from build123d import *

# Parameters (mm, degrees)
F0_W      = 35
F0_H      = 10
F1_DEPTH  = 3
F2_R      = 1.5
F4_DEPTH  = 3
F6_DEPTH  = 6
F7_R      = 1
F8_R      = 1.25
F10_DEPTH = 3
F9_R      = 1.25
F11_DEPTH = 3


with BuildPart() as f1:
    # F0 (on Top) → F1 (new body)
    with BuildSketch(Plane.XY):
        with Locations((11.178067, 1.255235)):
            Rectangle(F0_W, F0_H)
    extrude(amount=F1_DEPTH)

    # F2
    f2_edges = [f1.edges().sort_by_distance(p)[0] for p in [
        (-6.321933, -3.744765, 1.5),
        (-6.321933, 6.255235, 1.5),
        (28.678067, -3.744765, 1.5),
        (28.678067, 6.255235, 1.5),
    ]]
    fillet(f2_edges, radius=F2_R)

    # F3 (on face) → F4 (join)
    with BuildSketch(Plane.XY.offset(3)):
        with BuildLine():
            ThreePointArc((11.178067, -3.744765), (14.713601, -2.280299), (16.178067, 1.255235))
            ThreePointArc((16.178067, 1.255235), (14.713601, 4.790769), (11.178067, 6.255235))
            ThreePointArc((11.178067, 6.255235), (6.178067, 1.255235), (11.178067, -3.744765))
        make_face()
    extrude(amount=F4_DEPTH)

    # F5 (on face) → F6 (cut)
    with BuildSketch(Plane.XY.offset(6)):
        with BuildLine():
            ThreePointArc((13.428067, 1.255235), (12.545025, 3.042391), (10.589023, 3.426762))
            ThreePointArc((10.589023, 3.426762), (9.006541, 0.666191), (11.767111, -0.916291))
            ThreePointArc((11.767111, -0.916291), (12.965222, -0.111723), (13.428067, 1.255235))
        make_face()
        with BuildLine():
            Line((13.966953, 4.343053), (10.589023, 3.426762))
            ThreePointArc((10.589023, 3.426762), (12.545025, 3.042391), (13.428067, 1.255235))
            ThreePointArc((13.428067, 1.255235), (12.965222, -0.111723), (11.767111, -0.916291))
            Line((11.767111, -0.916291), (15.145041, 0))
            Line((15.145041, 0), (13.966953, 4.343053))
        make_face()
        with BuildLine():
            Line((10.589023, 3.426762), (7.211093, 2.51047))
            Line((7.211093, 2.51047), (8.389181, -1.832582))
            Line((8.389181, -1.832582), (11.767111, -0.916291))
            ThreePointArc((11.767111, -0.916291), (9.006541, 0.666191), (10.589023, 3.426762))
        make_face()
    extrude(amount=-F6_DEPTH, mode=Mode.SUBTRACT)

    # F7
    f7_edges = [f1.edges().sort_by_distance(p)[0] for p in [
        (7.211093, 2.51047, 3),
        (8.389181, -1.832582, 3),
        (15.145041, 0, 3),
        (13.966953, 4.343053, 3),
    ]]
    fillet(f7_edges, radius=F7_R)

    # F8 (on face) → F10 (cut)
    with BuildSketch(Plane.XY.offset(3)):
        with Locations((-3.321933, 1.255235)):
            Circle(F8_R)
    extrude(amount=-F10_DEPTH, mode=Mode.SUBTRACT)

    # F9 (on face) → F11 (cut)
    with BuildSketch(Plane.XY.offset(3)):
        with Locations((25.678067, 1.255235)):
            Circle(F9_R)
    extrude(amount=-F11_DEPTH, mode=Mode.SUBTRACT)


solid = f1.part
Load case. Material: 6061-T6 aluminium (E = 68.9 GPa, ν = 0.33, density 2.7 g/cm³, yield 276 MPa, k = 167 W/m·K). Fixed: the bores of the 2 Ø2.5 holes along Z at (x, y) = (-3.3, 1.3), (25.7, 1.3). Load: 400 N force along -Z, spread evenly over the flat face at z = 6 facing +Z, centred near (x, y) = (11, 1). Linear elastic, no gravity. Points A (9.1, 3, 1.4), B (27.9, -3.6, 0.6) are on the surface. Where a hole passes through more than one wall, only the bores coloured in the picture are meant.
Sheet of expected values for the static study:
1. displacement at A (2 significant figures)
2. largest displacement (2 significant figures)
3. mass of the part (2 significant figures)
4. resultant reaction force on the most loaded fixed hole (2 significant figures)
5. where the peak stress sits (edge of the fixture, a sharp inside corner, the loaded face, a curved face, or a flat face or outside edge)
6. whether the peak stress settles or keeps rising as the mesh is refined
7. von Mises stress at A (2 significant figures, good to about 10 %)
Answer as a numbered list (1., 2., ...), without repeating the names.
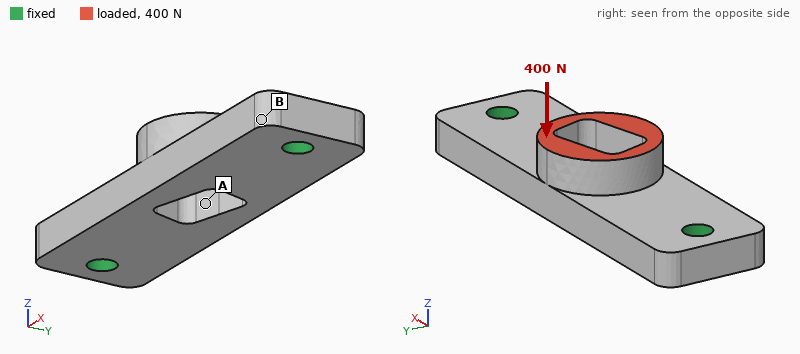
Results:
1. 25 µm
2. 28 µm
3. 2.9 g
4. 220 N
5. edge of the fixture
6. keeps rising
7. 30 MPa
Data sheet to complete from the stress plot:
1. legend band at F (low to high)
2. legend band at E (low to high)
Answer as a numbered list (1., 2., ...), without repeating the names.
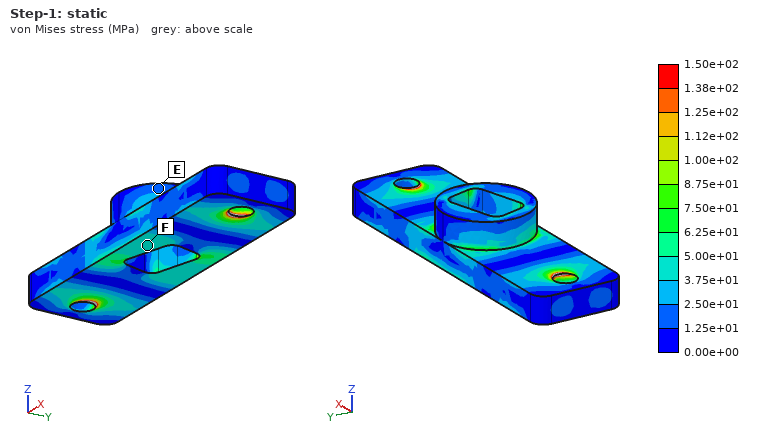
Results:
1. 3.75e+01 to 5.00e+01 MPa
2. 1.25e+01 to 2.50e+01 MPa
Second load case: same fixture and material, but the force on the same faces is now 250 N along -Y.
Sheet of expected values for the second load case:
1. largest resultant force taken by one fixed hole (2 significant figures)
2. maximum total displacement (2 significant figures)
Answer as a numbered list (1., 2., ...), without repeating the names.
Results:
1. 130 N
2. 27 µm
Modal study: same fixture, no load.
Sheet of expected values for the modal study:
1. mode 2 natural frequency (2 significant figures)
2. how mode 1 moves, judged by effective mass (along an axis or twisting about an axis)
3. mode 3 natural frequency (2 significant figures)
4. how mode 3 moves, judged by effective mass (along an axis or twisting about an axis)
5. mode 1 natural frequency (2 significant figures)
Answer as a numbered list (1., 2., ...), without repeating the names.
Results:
1. 22 kHz
2. along Z
3. 31 kHz
4. along Y
5. 18 kHz
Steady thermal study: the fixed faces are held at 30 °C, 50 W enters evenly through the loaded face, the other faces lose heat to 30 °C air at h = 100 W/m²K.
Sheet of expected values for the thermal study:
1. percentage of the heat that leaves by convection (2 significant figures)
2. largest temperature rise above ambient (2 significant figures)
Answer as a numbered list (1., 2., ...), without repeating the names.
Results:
1. 6.9 %
2. 80 K
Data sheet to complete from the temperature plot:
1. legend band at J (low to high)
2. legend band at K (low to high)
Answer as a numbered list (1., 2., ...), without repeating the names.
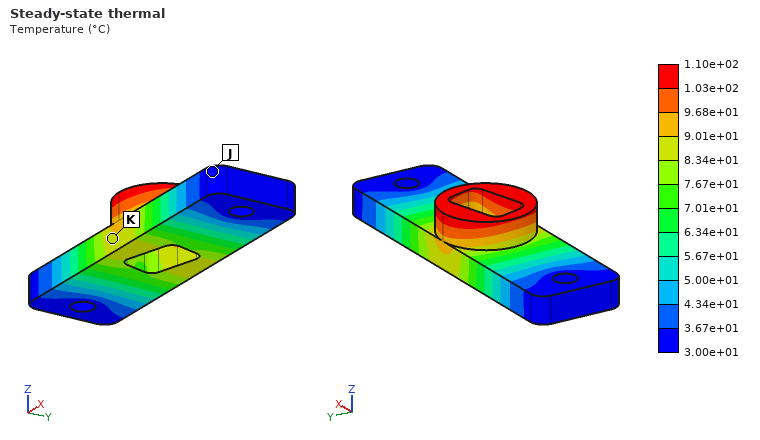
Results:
1. 3.00e+01 to 3.67e+01 °C
2. 8.34e+01 to 9.01e+01 °C
